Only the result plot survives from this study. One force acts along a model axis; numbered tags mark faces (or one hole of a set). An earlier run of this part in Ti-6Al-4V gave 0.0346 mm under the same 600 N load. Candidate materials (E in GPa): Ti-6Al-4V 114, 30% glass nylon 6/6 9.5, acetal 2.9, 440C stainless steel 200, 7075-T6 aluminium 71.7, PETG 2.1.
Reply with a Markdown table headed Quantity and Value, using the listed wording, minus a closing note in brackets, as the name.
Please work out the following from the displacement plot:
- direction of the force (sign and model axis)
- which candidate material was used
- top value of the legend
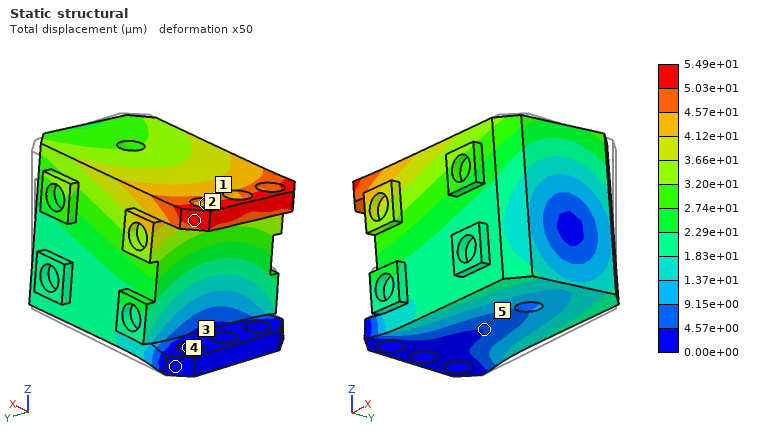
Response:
| Quantity | Value |
|---|---|
| direction of the force | -Y |
| which candidate material was used | 7075-T6 aluminium |
| top value of the legend | 5.49e+01 µm |
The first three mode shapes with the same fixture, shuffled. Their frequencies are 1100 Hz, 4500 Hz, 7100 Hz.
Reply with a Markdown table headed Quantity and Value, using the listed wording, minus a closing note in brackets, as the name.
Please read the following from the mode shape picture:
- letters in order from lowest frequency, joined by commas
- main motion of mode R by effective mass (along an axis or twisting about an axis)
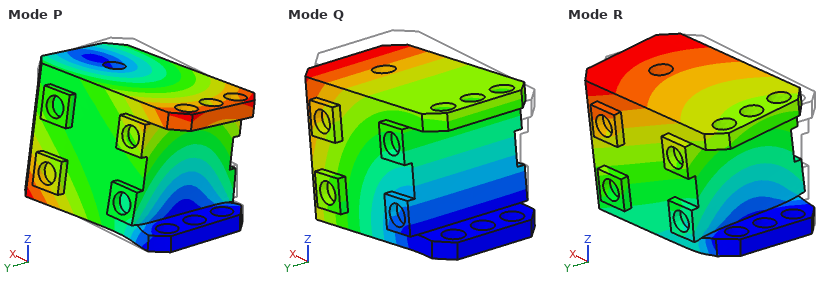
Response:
| Quantity | Value |
|---|---|
| letters in order from lowest frequency, joined by commas | Q, R, P |
| main motion of mode R by effective mass | along Y |
